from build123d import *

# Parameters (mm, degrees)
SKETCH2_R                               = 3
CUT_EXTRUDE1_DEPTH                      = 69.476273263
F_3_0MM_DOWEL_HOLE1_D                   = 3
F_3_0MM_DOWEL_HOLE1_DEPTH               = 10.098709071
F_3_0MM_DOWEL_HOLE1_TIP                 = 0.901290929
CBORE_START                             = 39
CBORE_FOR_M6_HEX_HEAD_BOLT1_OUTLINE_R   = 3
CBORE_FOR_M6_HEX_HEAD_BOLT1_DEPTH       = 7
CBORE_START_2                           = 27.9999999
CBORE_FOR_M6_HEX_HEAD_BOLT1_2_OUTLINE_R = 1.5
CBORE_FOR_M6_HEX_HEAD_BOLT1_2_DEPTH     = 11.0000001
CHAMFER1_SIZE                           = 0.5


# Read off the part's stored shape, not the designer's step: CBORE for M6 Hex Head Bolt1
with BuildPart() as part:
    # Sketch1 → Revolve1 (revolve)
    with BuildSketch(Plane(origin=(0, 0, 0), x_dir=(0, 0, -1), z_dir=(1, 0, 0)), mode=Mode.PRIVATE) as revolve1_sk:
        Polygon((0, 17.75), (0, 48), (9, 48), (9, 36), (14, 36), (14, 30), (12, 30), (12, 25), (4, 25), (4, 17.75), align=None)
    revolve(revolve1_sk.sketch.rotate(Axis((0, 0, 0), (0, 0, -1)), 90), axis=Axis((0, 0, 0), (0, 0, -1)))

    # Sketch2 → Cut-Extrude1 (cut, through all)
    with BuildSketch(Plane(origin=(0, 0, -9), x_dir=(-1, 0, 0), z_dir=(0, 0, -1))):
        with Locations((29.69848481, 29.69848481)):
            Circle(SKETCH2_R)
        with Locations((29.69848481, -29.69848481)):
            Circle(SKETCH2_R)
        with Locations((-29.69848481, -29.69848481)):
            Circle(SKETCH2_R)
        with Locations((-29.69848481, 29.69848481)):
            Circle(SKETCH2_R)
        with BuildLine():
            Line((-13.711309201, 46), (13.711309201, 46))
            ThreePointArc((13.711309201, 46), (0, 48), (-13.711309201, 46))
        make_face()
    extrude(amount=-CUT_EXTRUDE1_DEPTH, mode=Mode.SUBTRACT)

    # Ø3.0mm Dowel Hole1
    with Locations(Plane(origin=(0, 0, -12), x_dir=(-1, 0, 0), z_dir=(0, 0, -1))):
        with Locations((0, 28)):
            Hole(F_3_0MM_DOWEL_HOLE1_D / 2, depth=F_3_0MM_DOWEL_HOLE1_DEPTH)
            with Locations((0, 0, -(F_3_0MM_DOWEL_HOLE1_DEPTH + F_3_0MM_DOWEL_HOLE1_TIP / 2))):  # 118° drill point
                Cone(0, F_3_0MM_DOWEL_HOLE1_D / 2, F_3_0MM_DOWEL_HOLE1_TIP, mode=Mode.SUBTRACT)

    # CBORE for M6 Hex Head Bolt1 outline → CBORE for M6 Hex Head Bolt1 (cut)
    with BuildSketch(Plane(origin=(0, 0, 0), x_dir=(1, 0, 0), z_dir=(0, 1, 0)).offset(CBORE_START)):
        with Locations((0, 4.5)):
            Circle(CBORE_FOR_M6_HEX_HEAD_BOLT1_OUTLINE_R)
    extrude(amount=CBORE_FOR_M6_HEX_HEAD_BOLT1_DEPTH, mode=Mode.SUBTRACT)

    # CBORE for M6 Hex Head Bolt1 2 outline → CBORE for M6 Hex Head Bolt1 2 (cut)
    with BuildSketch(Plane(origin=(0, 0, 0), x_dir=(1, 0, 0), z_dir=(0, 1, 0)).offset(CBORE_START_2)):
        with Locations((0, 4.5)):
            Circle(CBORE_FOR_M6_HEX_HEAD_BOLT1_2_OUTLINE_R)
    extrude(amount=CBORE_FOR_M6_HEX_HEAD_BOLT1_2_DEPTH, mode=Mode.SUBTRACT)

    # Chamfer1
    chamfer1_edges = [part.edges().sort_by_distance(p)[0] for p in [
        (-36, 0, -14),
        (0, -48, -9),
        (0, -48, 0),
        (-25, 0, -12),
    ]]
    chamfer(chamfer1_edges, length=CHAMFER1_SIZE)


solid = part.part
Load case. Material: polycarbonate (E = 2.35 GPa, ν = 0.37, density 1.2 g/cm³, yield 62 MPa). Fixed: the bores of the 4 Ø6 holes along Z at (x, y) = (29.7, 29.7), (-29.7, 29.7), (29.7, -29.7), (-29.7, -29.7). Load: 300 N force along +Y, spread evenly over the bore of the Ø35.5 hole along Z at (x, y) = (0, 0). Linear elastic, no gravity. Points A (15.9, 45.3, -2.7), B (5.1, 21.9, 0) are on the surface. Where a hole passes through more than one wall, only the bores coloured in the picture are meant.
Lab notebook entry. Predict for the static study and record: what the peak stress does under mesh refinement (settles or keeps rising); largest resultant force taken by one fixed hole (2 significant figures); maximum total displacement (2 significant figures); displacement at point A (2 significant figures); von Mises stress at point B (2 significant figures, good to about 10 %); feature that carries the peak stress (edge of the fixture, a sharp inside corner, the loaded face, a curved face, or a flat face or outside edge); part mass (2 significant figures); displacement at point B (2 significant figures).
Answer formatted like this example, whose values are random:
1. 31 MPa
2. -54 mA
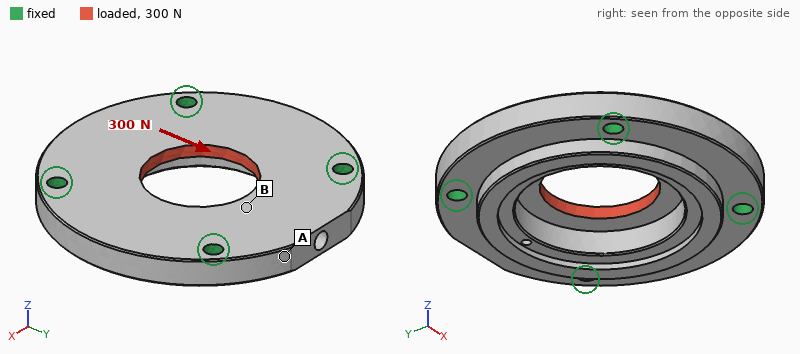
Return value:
1. keeps rising
2. 76 N
3. 14 µm
4. 6.7 µm
5. 0.60 MPa
6. edge of the fixture
7. 70 g
8. 12 µm
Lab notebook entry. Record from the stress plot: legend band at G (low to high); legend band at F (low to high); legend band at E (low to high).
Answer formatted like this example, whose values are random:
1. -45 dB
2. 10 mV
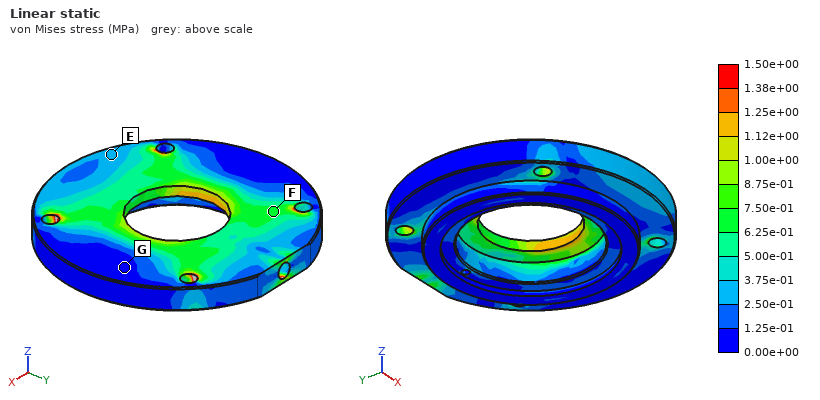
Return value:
1. 0.00e+00 to 1.25e-01 MPa
2. 6.25e-01 to 7.50e-01 MPa
3. 2.50e-01 to 3.75e-01 MPa
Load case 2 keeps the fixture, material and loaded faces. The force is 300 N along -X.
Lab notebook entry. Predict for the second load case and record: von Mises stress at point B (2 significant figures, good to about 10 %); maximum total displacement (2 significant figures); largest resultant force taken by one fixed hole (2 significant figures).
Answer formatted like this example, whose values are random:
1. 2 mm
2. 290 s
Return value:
1. 0.62 MPa
2. 14 µm
3. 76 N
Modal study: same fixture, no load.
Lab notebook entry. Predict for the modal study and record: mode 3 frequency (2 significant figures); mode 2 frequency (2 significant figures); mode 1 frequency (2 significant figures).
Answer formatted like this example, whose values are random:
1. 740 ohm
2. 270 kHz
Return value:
1. 3100 Hz
2. 3100 Hz
3. 2800 Hz
